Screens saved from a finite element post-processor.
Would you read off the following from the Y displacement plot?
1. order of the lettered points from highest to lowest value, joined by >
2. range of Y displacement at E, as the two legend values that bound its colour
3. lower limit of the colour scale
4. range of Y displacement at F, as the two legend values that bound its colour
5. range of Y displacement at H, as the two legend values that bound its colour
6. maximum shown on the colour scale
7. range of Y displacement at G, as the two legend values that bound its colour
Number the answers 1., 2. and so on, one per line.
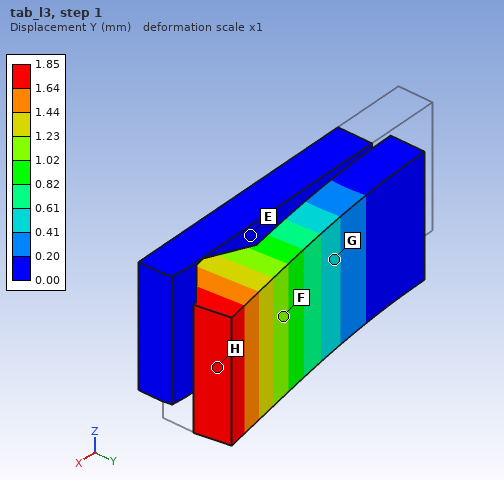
1. H > F > G > E
2. 0.00 to 0.20 mm
3. 0.00 mm
4. 1.02 to 1.23 mm
5. 1.64 to 1.85 mm
6. 1.85 mm
7. 0.41 to 0.61 mm
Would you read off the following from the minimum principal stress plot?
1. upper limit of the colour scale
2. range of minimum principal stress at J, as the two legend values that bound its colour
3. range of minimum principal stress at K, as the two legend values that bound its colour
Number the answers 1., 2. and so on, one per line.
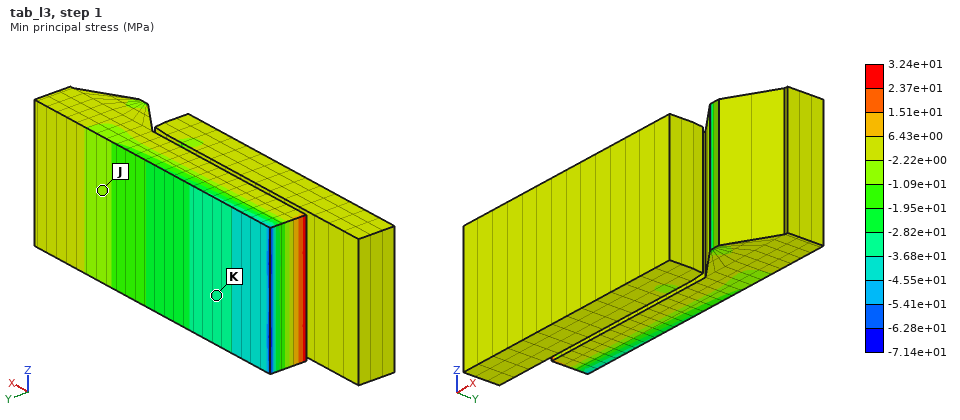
1. 3.24e+01 MPa
2. -1.09e+01 to -2.22e+00 MPa
3. -3.68e+01 to -2.82e+01 MPa
